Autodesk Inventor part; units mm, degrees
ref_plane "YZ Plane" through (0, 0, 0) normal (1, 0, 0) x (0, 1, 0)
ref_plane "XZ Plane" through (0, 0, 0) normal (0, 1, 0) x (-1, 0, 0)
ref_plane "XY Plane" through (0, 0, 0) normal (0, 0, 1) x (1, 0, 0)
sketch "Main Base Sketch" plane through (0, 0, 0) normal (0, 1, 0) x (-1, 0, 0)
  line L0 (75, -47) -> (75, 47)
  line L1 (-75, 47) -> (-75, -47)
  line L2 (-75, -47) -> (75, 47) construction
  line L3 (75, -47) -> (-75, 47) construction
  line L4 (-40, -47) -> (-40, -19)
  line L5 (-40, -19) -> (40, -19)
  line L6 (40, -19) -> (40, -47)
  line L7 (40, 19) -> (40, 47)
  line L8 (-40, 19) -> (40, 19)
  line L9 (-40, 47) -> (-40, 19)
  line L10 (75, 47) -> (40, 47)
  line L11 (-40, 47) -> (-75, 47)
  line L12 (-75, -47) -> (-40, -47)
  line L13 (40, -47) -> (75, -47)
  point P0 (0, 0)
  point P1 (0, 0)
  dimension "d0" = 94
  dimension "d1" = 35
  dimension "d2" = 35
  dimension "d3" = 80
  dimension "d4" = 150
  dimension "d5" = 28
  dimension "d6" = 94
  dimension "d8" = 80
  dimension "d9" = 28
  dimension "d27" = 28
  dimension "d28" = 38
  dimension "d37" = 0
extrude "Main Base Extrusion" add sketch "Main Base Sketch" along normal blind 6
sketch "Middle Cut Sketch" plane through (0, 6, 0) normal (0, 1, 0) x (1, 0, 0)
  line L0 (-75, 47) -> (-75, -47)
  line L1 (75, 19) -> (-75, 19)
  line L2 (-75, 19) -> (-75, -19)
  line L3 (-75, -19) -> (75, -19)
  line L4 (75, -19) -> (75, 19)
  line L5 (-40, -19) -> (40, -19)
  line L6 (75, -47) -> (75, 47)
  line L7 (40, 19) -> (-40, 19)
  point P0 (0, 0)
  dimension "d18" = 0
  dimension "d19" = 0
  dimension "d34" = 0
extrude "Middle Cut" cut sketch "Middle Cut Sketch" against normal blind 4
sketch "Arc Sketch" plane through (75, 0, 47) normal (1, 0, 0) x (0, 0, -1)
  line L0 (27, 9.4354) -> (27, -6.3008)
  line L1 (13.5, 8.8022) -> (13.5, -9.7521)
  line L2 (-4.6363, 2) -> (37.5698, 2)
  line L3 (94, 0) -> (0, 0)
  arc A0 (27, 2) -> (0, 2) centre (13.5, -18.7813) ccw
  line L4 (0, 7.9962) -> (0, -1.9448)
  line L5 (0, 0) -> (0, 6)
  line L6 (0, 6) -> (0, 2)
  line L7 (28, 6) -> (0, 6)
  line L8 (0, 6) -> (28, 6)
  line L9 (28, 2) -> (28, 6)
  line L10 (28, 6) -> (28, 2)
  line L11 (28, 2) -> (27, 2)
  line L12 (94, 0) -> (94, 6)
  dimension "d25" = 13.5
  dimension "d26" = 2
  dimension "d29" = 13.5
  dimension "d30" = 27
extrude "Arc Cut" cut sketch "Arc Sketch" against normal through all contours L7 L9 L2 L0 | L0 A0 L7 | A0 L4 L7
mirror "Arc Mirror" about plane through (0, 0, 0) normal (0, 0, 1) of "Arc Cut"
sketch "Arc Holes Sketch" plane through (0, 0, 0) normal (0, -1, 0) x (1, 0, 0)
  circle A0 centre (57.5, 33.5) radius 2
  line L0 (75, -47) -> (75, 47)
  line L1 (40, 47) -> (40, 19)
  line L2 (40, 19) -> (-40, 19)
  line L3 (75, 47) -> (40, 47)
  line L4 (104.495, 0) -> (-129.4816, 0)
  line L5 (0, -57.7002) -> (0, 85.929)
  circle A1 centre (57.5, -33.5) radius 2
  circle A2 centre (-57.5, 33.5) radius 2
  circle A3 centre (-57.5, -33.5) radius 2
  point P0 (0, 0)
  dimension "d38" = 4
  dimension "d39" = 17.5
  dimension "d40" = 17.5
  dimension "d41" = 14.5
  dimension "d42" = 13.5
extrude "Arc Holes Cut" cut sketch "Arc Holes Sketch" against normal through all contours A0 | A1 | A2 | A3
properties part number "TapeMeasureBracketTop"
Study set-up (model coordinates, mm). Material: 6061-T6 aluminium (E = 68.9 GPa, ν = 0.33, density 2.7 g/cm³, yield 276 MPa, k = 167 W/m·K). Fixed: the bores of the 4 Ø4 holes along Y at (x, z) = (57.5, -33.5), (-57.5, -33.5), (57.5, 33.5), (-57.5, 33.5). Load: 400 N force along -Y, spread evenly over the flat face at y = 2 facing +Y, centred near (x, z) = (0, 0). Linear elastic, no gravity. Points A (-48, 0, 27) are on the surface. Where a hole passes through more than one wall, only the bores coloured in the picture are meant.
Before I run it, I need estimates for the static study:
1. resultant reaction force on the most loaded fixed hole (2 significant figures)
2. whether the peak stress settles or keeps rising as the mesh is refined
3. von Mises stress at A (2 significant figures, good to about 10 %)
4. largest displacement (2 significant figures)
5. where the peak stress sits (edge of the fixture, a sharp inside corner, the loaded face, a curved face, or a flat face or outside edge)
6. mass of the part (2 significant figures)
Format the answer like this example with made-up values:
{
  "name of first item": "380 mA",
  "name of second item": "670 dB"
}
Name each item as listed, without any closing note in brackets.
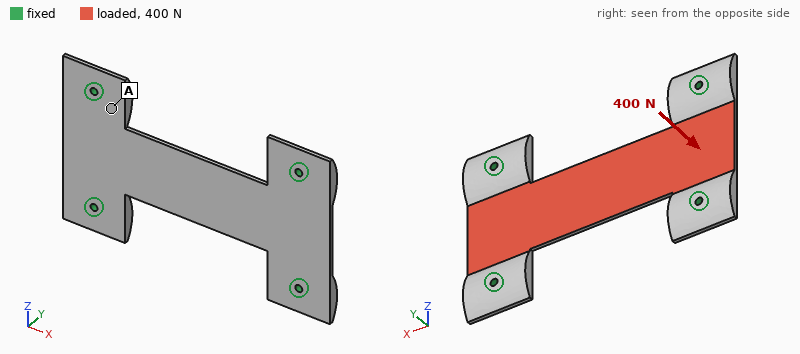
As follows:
{
  "resultant reaction force on the most loaded fixed hole": "210 N",
  "whether the peak stress settles or keeps rising as the mesh is refined": "keeps rising",
  "von Mises stress at A": "13 MPa",
  "largest displacement": "0.37 mm",
  "where the peak stress sits": "a sharp inside corner",
  "mass of the part": "79 g"
}
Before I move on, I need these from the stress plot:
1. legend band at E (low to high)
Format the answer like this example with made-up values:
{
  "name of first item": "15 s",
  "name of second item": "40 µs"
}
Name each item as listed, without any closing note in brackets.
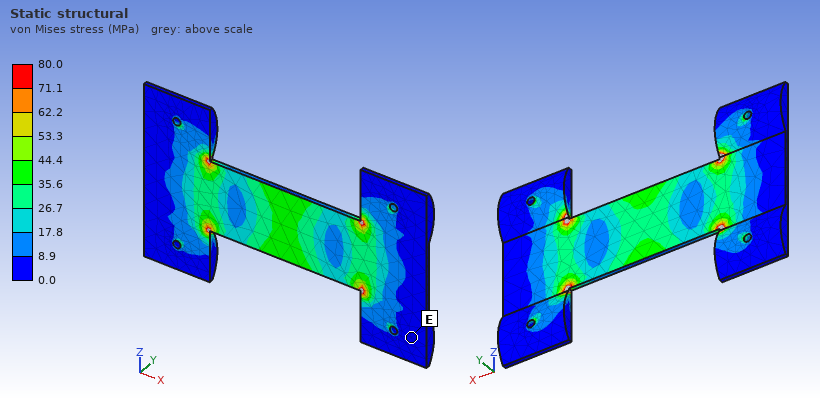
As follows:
{
  "legend band at E": "0.0 to 8.9 MPa"
}
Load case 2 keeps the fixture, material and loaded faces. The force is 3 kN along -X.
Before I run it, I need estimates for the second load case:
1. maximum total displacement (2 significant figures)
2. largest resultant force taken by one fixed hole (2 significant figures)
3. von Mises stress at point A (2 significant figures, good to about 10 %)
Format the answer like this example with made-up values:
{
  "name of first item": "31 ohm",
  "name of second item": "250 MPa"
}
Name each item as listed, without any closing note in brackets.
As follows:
{
  "maximum total displacement": "21 µm",
  "largest resultant force taken by one fixed hole": "760 N",
  "von Mises stress at point A": "16 MPa"
}
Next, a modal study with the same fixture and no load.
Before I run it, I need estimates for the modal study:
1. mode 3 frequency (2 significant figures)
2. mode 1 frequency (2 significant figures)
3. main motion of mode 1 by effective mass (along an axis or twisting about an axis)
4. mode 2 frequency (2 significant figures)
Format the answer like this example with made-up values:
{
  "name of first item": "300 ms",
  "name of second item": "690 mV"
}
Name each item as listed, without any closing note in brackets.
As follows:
{
  "mode 3 frequency": "2800 Hz",
  "mode 1 frequency": "1100 Hz",
  "main motion of mode 1 by effective mass": "along Y",
  "mode 2 frequency": "2300 Hz"
}
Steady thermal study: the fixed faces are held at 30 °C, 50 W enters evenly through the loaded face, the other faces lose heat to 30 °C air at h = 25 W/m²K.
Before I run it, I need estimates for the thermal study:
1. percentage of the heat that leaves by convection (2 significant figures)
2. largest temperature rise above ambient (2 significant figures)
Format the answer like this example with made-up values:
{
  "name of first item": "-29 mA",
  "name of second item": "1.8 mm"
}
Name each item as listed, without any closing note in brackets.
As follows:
{
  "percentage of the heat that leaves by convection": "9.4 %",
  "largest temperature rise above ambient": "40 K"
}
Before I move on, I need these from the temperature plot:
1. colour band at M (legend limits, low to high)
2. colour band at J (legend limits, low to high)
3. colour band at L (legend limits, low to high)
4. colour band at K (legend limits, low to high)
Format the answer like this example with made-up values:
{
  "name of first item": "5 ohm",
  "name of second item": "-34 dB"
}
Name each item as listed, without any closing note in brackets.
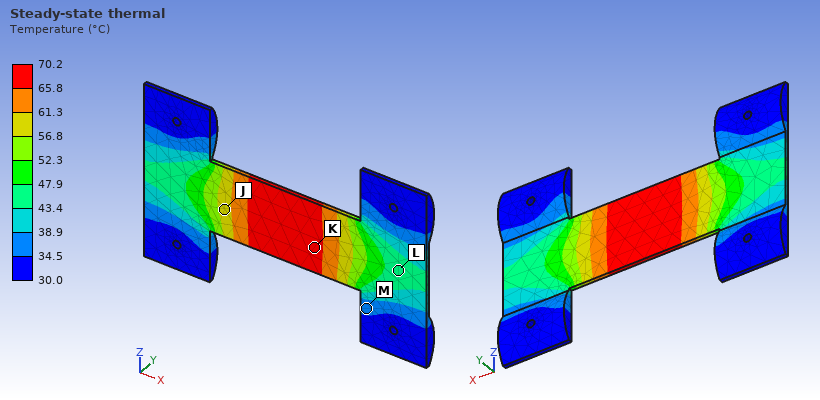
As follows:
{
  "colour band at M": "34.5 to 38.9 °C",
  "colour band at J": "56.8 to 61.3 °C",
  "colour band at L": "43.4 to 47.9 °C",
  "colour band at K": "65.8 to 70.2 °C"
}
